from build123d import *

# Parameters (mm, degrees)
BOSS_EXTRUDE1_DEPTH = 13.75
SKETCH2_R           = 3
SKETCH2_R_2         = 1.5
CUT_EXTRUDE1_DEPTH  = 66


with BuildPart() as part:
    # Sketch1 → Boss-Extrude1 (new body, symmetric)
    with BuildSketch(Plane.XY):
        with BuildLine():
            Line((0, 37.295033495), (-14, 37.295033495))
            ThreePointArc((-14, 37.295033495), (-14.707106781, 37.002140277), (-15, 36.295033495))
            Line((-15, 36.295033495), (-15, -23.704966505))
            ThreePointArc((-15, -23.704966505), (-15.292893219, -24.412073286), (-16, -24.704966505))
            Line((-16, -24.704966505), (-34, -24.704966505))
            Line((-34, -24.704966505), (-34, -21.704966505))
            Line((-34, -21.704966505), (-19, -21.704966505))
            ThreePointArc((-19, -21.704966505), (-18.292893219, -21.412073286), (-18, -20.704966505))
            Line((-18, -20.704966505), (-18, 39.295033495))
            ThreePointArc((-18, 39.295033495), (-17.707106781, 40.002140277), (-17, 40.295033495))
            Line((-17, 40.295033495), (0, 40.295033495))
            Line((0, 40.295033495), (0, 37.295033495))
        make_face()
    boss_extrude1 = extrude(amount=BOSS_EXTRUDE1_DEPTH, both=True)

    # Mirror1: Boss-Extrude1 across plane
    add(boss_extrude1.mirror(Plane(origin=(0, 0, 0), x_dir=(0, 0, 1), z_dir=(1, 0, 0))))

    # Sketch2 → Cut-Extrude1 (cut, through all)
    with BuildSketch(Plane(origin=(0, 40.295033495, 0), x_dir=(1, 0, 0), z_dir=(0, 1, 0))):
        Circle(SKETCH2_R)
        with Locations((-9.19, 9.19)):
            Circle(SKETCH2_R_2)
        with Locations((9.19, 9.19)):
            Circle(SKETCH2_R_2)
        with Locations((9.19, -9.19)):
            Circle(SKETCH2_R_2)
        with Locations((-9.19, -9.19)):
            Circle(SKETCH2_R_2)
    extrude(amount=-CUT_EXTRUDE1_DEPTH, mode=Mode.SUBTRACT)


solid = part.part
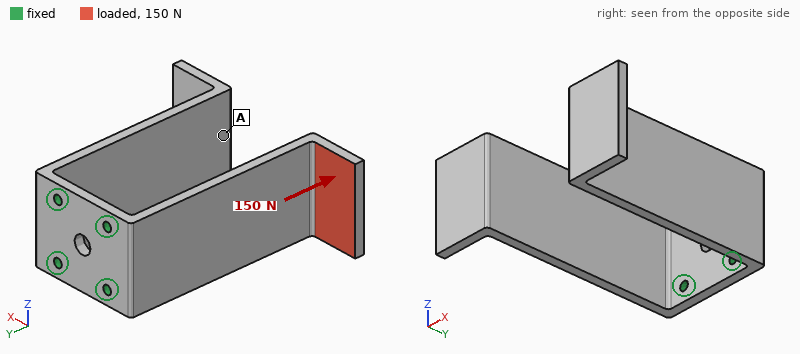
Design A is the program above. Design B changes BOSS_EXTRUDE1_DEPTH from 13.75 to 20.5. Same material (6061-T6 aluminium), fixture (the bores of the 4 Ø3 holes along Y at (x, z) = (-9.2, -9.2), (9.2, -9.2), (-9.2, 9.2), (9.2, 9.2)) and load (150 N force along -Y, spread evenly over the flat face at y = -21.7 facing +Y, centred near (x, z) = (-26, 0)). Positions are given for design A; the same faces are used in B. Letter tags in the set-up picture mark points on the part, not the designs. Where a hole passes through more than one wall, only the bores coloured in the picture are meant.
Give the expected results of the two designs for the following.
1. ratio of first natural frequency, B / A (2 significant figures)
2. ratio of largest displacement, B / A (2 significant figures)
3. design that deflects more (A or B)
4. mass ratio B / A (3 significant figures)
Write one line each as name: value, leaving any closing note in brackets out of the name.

ratio of first natural frequency, B / A: 0.99
ratio of largest displacement, B / A: 0.68
design that deflects more: A
mass ratio B / A: 1.50
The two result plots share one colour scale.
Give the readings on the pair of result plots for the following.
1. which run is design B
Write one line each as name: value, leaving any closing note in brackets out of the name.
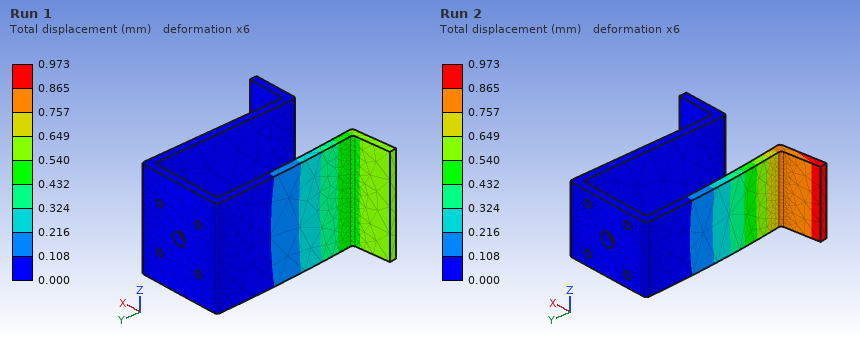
which run is design B: Run 1
